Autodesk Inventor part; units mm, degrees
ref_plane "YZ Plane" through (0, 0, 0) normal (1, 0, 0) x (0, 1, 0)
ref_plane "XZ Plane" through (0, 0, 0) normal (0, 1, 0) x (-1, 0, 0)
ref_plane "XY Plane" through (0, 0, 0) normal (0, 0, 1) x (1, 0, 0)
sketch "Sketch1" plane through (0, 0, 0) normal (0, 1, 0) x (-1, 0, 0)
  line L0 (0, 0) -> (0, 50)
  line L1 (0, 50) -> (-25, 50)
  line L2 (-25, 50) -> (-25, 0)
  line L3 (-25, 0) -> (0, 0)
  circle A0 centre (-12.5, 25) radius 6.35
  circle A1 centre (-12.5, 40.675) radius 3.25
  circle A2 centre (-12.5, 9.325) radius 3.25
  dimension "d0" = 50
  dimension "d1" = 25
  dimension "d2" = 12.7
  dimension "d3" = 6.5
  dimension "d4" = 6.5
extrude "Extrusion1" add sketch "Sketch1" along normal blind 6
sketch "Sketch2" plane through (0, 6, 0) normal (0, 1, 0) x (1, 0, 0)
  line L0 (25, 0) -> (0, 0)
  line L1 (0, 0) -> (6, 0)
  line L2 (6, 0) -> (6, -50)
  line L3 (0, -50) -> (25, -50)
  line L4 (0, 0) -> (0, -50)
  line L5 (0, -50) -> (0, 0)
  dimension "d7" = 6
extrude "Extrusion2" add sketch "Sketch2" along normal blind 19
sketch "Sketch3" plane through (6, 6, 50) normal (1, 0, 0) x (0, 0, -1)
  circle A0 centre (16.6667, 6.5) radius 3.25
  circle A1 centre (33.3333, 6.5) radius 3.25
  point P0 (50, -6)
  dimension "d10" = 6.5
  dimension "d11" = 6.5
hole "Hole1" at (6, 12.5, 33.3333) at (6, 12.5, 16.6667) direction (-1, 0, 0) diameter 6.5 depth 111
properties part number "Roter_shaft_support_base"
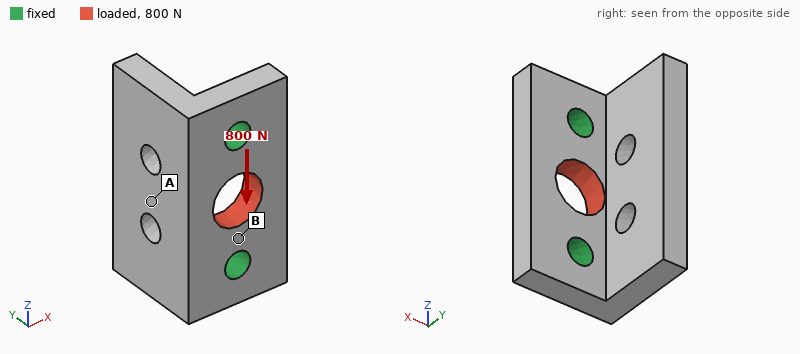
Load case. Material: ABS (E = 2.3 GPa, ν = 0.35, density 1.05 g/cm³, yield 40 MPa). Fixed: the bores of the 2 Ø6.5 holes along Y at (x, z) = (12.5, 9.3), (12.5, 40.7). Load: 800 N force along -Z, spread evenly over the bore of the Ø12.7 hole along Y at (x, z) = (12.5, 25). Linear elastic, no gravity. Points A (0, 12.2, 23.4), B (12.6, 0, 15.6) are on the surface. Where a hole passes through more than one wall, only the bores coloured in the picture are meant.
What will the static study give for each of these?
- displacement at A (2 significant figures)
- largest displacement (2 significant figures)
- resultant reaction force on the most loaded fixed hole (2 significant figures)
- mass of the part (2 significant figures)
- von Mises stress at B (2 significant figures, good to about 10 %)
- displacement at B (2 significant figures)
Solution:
11 µm
27 µm
400 N
12 g
4.8 MPa
7.2 µm
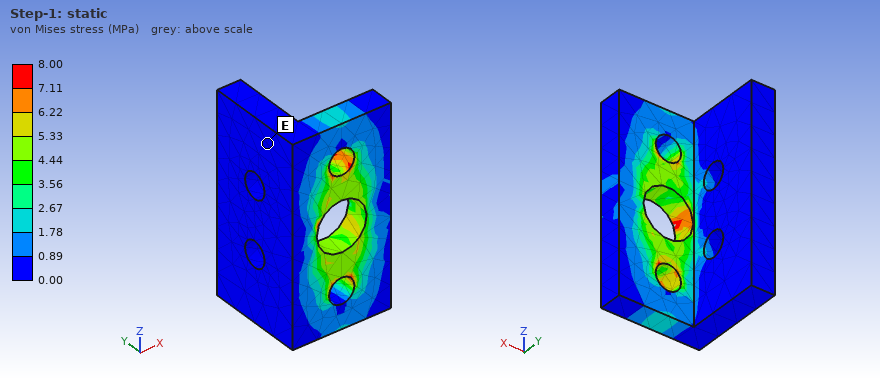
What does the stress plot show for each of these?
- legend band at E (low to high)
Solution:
0.00 to 0.89 MPa
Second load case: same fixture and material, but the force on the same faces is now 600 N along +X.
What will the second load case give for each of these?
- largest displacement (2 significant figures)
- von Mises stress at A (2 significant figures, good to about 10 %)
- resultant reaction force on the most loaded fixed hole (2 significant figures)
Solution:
46 µm
1.1 MPa
300 N
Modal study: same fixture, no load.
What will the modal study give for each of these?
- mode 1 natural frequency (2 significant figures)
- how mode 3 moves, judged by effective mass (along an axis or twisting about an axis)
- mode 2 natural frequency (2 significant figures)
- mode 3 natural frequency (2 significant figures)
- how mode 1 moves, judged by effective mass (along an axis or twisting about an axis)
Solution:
1800 Hz
along Z
2900 Hz
4700 Hz
along X
